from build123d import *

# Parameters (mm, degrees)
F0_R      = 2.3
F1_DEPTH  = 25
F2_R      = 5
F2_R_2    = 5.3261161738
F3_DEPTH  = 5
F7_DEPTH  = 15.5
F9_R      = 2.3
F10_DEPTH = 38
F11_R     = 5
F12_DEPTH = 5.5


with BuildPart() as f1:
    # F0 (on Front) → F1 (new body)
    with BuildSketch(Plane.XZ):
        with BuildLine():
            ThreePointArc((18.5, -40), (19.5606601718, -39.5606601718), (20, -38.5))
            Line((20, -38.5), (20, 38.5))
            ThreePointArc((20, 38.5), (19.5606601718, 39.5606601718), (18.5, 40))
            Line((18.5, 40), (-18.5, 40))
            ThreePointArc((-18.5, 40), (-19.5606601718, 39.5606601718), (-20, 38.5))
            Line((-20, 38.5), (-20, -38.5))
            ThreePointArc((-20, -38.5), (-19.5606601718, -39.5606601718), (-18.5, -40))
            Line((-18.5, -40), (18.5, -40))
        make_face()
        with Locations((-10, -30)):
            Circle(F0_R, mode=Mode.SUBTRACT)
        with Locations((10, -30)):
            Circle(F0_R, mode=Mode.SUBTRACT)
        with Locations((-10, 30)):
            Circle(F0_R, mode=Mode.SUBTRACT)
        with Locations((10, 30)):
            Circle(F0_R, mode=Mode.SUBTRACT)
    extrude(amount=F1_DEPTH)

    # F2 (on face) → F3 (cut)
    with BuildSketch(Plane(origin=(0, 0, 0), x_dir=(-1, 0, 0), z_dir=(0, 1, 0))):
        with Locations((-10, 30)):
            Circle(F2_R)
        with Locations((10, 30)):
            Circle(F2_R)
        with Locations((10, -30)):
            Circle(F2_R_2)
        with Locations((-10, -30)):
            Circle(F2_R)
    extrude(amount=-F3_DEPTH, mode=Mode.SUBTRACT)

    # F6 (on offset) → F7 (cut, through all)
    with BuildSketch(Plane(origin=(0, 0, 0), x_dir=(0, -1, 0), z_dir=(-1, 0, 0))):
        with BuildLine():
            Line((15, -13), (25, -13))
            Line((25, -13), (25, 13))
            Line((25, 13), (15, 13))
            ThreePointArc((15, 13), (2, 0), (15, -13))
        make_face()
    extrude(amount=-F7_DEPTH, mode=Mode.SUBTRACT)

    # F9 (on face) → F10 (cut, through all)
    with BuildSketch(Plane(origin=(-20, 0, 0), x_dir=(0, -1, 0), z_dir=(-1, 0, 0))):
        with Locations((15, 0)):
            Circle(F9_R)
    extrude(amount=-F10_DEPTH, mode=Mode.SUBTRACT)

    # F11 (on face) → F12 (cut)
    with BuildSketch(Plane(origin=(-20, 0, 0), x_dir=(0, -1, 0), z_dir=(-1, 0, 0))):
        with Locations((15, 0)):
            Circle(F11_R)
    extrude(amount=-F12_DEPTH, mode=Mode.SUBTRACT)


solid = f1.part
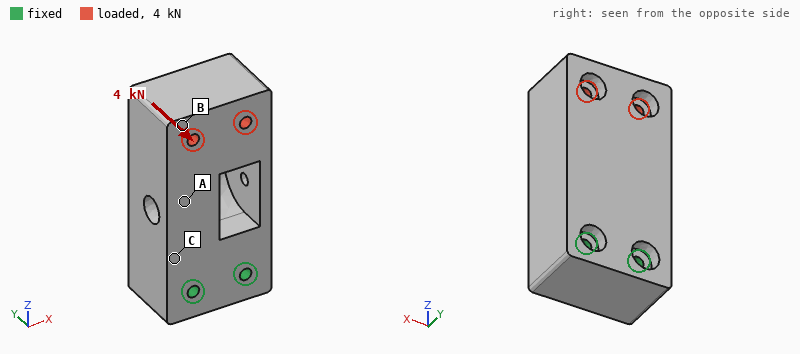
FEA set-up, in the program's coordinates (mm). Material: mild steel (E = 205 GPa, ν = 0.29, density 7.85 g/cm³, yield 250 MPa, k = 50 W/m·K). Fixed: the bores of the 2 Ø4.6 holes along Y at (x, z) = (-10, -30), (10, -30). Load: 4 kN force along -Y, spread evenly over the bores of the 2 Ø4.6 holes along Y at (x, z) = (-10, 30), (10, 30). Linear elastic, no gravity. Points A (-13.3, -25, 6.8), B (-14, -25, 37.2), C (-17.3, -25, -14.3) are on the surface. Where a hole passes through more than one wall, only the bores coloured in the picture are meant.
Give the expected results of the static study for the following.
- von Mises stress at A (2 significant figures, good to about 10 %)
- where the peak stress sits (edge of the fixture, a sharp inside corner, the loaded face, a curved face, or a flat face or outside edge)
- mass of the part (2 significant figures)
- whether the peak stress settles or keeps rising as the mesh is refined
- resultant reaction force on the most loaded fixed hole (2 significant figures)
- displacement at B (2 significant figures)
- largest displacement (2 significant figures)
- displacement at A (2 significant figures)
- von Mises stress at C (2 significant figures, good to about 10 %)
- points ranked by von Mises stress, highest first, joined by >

29 MPa
edge of the fixture
530 g
keeps rising
2.0 kN
60 µm
65 µm
28 µm
53 MPa
C > A > B
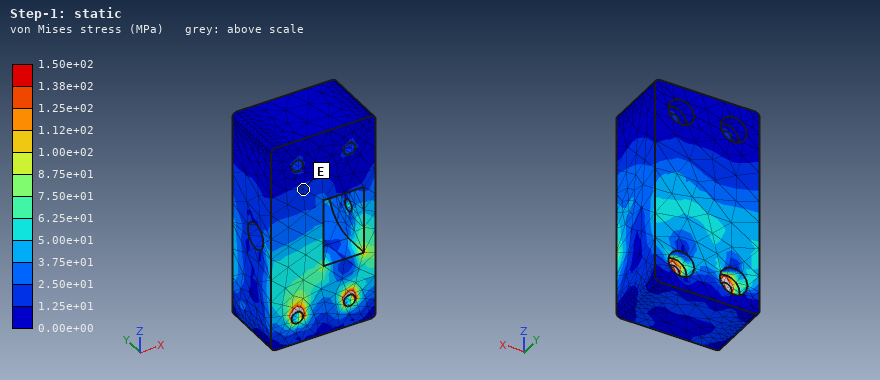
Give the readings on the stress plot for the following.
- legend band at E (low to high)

1.25e+01 to 2.50e+01 MPa
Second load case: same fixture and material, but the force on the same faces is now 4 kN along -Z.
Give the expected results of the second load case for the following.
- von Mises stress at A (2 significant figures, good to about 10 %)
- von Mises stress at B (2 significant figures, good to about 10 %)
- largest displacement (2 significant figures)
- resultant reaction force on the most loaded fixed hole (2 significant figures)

10 MPa
2.8 MPa
5.4 µm
2.0 kN
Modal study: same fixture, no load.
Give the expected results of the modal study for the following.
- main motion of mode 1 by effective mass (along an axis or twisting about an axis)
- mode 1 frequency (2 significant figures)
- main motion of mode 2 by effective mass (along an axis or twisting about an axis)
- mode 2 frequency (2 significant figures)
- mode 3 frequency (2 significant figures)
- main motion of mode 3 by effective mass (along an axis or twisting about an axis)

along Y
3100 Hz
along X
4200 Hz
8100 Hz
twisting about Z
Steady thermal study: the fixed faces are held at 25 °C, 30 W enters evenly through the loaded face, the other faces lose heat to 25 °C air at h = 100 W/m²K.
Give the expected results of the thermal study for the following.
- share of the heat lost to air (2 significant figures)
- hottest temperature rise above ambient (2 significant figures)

60 %
29 K
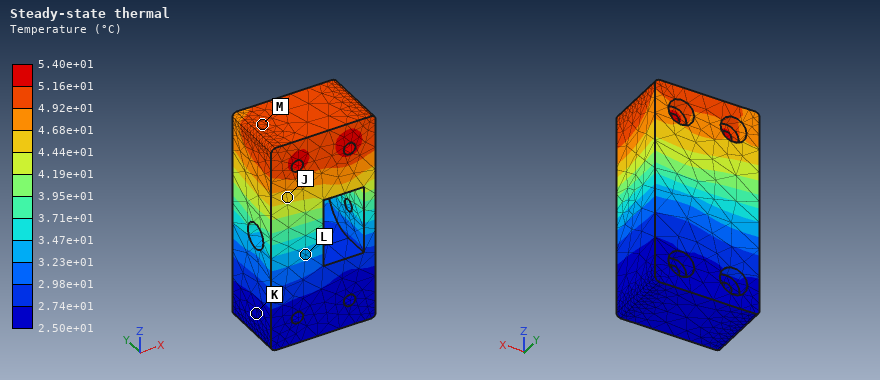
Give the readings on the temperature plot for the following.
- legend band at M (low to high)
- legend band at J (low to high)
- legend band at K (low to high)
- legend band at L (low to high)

4.92e+01 to 5.16e+01 °C
4.44e+01 to 4.68e+01 °C
2.50e+01 to 2.74e+01 °C
3.23e+01 to 3.47e+01 °C
